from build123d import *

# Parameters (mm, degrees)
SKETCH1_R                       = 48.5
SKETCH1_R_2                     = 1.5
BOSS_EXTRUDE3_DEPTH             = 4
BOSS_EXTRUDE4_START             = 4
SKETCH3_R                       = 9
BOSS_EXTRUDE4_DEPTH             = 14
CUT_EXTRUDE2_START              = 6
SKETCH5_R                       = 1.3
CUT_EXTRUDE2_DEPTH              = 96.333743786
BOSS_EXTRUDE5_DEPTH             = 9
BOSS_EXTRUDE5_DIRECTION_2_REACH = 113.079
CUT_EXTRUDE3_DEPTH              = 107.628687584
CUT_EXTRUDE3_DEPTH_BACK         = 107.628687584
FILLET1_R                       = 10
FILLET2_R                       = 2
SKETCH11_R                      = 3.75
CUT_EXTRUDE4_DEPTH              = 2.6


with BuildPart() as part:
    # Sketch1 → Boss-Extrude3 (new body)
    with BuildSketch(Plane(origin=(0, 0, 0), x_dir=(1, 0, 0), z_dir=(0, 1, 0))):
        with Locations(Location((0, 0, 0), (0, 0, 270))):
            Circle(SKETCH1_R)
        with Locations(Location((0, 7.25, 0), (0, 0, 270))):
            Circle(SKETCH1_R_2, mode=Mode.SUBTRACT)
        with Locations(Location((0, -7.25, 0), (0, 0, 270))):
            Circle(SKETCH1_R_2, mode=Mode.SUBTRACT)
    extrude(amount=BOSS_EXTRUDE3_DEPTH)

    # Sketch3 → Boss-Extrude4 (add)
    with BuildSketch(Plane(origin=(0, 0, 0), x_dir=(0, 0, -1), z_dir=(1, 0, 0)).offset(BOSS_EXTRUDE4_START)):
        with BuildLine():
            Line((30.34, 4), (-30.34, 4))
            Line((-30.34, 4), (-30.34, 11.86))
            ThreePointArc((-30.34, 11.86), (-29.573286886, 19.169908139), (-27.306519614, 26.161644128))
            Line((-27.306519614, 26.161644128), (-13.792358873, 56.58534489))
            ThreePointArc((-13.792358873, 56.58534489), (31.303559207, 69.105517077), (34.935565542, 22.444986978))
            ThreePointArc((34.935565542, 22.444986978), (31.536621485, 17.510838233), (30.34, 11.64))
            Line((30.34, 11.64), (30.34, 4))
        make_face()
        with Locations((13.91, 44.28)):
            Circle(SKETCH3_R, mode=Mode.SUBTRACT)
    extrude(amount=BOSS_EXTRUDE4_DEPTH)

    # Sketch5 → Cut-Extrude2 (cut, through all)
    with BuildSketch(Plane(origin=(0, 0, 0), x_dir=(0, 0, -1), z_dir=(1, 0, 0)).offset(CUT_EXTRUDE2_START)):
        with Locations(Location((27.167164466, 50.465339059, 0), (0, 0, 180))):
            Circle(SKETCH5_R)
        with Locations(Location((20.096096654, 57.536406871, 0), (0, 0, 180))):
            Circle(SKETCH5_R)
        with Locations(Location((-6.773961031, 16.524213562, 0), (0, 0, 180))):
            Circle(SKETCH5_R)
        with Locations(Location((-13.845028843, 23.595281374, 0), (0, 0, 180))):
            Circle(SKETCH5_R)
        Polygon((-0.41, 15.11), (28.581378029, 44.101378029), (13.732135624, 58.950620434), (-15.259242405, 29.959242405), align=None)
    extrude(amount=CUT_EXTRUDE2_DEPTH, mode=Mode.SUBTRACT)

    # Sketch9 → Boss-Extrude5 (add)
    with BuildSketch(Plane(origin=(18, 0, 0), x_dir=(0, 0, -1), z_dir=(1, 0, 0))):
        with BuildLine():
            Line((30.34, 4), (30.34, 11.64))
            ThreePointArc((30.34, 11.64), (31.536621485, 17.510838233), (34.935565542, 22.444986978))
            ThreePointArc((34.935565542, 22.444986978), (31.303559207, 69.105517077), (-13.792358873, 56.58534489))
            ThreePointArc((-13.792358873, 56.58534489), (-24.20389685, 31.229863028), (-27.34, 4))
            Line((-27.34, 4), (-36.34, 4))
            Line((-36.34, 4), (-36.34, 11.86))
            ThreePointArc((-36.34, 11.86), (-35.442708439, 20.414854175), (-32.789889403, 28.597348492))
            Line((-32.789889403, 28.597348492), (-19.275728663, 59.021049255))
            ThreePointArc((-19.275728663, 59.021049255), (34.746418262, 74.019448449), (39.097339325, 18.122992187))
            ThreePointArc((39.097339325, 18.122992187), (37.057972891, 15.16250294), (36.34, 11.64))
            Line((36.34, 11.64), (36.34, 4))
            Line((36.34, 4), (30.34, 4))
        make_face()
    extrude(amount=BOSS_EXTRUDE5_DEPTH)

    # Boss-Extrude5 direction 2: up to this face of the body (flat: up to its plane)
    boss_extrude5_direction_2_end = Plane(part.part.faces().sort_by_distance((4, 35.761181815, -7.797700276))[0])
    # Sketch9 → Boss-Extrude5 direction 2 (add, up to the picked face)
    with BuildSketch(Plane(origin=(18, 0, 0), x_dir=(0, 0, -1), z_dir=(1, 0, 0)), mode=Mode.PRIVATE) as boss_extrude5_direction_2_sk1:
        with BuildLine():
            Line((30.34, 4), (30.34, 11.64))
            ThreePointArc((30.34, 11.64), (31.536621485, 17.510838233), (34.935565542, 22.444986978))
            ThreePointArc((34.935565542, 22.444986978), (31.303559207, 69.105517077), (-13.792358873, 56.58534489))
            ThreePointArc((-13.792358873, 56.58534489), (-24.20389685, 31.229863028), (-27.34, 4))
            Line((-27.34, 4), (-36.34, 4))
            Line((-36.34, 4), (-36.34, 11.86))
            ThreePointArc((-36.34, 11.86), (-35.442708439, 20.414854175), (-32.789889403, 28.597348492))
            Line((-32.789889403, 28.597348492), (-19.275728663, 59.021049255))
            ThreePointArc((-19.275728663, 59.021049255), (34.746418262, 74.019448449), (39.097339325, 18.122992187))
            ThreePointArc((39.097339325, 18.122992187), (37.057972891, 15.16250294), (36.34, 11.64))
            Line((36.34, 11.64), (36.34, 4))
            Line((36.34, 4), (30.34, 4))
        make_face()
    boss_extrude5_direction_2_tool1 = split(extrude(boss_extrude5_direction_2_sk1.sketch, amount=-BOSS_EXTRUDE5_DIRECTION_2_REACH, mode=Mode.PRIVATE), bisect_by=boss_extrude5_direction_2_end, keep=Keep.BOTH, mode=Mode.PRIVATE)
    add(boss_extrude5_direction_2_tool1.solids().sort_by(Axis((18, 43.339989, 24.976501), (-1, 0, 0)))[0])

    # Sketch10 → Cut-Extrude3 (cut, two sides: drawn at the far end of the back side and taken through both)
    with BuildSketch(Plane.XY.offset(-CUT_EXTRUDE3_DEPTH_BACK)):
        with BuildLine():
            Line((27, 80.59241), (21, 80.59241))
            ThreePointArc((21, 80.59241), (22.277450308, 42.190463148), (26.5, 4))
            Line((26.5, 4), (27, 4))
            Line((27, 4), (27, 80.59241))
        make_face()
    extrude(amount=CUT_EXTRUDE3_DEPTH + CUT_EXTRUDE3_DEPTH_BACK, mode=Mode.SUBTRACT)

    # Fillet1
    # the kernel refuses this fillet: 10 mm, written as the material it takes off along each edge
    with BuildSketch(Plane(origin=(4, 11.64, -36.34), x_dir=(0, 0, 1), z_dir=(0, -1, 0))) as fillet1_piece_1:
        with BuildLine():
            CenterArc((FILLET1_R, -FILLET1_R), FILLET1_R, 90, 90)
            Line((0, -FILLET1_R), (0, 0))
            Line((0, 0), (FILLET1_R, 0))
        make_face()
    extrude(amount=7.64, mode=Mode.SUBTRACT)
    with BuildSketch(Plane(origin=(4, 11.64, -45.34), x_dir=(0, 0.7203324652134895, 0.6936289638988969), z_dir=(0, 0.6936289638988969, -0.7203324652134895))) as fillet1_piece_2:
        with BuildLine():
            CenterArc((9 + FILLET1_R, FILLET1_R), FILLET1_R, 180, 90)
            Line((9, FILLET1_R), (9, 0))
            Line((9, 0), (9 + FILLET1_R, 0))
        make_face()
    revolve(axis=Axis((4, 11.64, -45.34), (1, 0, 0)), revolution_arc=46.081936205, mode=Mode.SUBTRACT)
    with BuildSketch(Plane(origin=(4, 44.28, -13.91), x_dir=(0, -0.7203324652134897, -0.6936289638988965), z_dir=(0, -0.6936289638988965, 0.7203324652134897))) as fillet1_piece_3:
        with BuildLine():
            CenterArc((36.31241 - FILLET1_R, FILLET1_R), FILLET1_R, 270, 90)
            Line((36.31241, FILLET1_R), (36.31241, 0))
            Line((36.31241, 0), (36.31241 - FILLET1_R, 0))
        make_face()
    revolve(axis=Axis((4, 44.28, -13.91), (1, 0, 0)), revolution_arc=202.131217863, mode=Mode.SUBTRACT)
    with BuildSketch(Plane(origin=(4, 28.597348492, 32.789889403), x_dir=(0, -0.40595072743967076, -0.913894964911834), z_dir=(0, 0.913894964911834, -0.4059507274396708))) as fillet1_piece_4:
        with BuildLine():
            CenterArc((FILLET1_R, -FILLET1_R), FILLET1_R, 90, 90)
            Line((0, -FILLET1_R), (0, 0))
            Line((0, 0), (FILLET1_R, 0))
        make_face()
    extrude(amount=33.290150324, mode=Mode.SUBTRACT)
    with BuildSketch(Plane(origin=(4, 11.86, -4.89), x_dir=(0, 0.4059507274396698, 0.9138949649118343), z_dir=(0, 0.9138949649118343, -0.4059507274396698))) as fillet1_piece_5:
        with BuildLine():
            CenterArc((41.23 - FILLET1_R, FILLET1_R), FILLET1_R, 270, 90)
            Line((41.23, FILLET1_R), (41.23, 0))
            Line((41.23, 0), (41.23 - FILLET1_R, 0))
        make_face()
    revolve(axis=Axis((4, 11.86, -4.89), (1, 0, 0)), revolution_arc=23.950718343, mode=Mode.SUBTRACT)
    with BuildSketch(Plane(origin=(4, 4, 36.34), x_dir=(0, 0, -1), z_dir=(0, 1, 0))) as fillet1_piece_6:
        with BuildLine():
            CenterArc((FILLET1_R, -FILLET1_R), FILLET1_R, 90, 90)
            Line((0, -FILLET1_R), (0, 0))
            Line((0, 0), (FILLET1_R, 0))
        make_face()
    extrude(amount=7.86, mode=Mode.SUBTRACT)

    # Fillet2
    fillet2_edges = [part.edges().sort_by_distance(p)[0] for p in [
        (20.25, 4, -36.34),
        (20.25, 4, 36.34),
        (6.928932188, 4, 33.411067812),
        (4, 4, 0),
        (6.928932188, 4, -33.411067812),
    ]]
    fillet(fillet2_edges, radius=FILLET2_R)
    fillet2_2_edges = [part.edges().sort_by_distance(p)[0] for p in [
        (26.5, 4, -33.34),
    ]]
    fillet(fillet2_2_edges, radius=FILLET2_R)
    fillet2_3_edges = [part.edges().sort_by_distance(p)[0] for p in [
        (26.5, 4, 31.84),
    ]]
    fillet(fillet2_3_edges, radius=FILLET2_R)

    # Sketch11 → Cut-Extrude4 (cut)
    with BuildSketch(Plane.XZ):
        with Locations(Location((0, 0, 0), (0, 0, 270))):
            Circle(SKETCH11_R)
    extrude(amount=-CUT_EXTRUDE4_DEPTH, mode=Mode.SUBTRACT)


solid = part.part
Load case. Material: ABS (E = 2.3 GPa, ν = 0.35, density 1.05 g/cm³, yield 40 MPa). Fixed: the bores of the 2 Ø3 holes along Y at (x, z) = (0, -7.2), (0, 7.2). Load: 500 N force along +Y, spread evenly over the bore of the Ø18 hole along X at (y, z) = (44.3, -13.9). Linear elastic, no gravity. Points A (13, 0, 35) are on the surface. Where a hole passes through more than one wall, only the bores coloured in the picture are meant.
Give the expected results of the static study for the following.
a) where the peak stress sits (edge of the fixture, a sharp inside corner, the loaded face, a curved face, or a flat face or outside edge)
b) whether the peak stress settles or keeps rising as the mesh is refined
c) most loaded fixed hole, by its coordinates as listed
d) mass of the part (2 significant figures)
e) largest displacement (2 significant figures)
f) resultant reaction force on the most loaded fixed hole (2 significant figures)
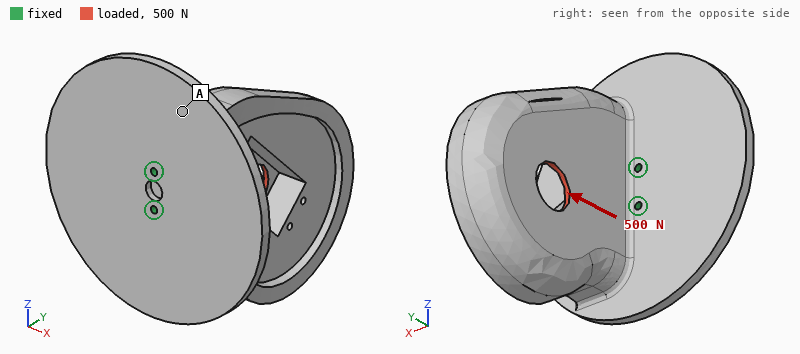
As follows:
edge of the fixture
keeps rising
(0, -7.2)
97 g
1.6 mm
620 N
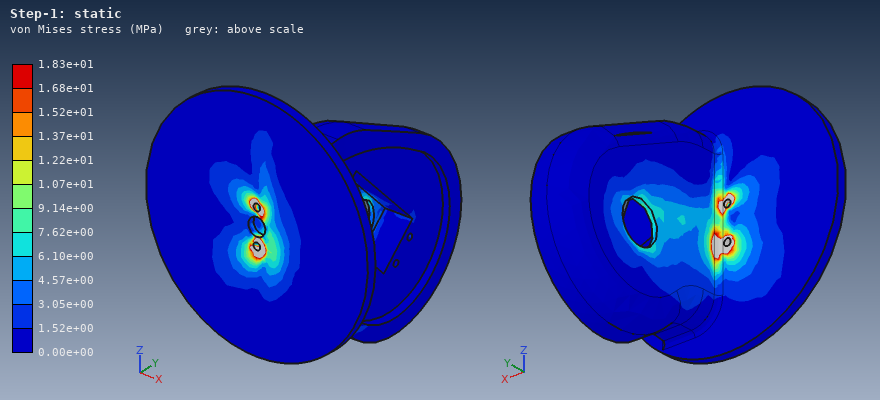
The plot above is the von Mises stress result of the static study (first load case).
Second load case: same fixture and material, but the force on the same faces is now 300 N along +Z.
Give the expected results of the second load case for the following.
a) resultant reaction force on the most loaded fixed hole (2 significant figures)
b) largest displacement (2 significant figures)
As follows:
700 N
1.8 mm
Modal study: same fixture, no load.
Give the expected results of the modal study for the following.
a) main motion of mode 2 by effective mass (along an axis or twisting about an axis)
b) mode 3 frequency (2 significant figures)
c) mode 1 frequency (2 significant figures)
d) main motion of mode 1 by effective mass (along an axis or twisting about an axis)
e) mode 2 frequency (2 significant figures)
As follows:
along Z
480 Hz
130 Hz
along X
290 Hz
